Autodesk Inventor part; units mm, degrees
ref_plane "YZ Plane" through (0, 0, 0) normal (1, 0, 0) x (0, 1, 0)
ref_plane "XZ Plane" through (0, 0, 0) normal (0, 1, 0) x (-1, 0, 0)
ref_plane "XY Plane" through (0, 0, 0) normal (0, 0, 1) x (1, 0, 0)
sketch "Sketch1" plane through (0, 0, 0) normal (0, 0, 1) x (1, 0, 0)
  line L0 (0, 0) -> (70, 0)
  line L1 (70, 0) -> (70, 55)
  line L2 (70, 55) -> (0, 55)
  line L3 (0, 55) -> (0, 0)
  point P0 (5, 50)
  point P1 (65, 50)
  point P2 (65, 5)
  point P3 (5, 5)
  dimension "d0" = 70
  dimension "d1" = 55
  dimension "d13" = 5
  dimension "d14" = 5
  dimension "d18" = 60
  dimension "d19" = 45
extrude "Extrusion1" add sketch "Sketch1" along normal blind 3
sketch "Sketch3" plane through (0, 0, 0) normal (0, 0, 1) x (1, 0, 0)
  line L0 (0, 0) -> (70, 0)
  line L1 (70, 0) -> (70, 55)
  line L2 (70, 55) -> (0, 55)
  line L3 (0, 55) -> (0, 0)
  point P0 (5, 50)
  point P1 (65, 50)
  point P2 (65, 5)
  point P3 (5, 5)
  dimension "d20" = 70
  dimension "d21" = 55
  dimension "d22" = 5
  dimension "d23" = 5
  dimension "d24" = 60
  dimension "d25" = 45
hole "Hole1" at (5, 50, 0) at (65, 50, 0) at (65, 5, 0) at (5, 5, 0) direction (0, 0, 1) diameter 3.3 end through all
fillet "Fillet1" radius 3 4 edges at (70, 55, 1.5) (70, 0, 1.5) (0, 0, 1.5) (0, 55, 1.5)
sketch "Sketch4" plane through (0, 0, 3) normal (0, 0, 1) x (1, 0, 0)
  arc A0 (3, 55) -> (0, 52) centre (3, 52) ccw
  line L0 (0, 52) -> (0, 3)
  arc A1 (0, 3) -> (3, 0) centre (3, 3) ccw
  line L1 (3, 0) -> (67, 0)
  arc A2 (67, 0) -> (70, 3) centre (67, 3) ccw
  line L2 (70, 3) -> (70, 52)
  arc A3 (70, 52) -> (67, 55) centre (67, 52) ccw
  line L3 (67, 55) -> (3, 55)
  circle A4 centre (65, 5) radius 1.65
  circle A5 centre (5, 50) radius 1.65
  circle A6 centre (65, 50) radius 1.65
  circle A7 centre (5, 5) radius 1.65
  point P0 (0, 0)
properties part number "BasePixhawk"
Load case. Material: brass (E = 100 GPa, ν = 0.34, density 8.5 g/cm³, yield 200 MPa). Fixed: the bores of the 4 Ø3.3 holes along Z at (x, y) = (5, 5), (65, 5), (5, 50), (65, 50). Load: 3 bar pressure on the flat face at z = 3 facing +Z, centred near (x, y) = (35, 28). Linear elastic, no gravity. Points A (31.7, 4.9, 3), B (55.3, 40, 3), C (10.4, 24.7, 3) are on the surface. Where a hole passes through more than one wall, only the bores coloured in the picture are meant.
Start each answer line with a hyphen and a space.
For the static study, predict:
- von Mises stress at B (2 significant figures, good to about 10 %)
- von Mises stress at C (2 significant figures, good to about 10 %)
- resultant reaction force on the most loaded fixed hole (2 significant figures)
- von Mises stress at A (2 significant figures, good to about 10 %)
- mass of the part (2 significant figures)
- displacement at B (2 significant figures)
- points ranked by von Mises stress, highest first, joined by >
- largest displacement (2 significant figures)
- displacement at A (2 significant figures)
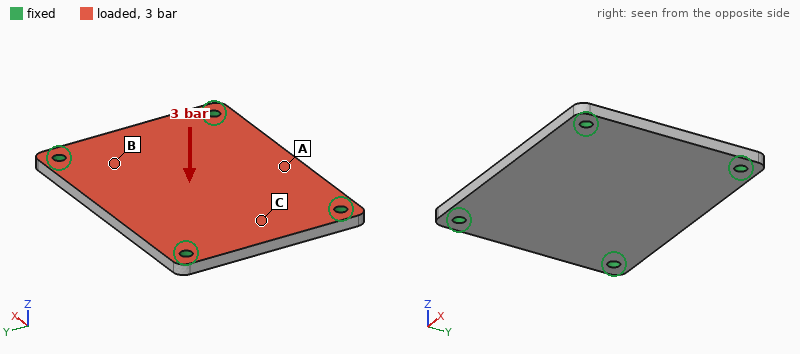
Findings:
- 11 MPa
- 22 MPa
- 290 N
- 36 MPa
- 97 g
- 34 µm
- A > C > B
- 75 µm
- 59 µm
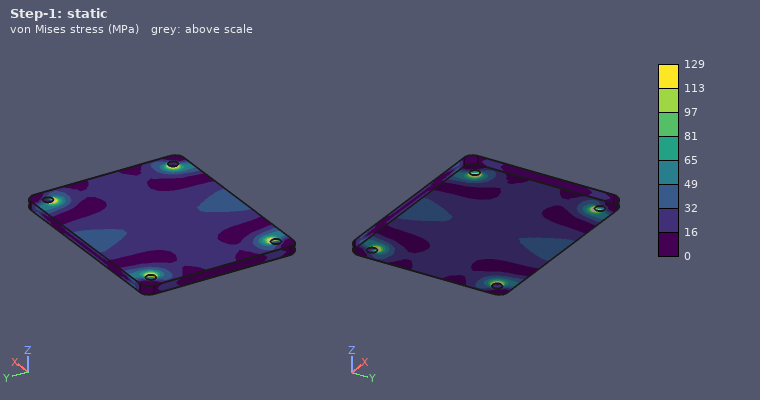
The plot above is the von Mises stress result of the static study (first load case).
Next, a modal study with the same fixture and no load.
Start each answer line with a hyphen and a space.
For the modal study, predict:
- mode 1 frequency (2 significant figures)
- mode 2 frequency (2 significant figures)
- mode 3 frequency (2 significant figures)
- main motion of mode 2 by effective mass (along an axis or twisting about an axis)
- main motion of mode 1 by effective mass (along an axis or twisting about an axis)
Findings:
- 2400 Hz
- 3600 Hz
- 5000 Hz
- twisting about X
- along Z
